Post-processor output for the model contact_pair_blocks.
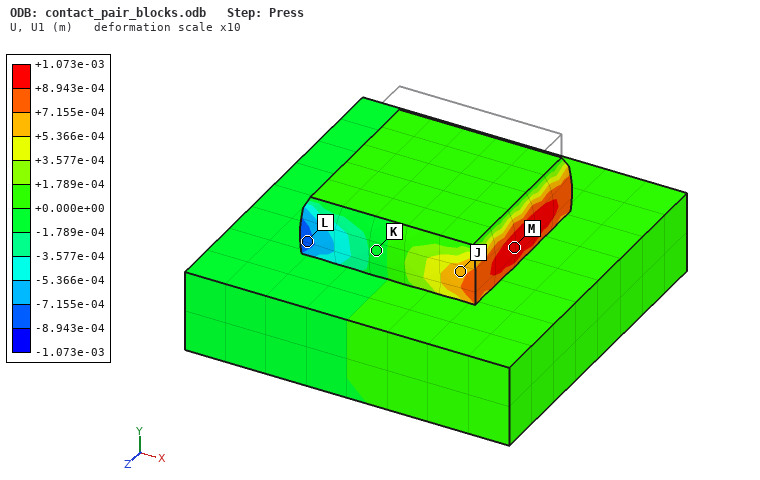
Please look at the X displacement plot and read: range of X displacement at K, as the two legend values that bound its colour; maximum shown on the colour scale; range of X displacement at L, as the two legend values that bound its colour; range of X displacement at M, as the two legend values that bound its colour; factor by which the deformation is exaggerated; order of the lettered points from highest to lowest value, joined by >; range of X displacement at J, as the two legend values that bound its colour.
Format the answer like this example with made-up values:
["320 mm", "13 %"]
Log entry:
["-1.789e-04 to +0.000e+00 m", "+1.073e-03 m", "-8.943e-04 to -7.155e-04 m", "+8.943e-04 to +1.073e-03 m", "10", "M > J > K > L", "+5.366e-04 to +7.155e-04 m"]
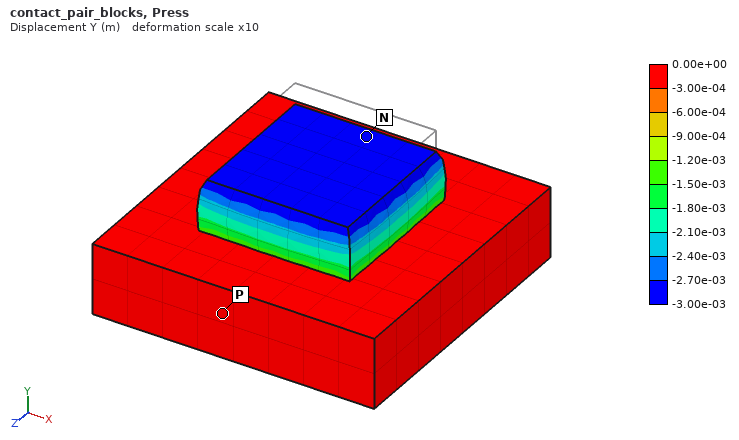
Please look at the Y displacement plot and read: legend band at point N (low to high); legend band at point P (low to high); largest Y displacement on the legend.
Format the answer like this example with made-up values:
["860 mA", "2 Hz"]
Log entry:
["-3.00e-03 to -2.70e-03 m", "-3.00e-04 to 0.00e+00 m", "0.00e+00 m"]
